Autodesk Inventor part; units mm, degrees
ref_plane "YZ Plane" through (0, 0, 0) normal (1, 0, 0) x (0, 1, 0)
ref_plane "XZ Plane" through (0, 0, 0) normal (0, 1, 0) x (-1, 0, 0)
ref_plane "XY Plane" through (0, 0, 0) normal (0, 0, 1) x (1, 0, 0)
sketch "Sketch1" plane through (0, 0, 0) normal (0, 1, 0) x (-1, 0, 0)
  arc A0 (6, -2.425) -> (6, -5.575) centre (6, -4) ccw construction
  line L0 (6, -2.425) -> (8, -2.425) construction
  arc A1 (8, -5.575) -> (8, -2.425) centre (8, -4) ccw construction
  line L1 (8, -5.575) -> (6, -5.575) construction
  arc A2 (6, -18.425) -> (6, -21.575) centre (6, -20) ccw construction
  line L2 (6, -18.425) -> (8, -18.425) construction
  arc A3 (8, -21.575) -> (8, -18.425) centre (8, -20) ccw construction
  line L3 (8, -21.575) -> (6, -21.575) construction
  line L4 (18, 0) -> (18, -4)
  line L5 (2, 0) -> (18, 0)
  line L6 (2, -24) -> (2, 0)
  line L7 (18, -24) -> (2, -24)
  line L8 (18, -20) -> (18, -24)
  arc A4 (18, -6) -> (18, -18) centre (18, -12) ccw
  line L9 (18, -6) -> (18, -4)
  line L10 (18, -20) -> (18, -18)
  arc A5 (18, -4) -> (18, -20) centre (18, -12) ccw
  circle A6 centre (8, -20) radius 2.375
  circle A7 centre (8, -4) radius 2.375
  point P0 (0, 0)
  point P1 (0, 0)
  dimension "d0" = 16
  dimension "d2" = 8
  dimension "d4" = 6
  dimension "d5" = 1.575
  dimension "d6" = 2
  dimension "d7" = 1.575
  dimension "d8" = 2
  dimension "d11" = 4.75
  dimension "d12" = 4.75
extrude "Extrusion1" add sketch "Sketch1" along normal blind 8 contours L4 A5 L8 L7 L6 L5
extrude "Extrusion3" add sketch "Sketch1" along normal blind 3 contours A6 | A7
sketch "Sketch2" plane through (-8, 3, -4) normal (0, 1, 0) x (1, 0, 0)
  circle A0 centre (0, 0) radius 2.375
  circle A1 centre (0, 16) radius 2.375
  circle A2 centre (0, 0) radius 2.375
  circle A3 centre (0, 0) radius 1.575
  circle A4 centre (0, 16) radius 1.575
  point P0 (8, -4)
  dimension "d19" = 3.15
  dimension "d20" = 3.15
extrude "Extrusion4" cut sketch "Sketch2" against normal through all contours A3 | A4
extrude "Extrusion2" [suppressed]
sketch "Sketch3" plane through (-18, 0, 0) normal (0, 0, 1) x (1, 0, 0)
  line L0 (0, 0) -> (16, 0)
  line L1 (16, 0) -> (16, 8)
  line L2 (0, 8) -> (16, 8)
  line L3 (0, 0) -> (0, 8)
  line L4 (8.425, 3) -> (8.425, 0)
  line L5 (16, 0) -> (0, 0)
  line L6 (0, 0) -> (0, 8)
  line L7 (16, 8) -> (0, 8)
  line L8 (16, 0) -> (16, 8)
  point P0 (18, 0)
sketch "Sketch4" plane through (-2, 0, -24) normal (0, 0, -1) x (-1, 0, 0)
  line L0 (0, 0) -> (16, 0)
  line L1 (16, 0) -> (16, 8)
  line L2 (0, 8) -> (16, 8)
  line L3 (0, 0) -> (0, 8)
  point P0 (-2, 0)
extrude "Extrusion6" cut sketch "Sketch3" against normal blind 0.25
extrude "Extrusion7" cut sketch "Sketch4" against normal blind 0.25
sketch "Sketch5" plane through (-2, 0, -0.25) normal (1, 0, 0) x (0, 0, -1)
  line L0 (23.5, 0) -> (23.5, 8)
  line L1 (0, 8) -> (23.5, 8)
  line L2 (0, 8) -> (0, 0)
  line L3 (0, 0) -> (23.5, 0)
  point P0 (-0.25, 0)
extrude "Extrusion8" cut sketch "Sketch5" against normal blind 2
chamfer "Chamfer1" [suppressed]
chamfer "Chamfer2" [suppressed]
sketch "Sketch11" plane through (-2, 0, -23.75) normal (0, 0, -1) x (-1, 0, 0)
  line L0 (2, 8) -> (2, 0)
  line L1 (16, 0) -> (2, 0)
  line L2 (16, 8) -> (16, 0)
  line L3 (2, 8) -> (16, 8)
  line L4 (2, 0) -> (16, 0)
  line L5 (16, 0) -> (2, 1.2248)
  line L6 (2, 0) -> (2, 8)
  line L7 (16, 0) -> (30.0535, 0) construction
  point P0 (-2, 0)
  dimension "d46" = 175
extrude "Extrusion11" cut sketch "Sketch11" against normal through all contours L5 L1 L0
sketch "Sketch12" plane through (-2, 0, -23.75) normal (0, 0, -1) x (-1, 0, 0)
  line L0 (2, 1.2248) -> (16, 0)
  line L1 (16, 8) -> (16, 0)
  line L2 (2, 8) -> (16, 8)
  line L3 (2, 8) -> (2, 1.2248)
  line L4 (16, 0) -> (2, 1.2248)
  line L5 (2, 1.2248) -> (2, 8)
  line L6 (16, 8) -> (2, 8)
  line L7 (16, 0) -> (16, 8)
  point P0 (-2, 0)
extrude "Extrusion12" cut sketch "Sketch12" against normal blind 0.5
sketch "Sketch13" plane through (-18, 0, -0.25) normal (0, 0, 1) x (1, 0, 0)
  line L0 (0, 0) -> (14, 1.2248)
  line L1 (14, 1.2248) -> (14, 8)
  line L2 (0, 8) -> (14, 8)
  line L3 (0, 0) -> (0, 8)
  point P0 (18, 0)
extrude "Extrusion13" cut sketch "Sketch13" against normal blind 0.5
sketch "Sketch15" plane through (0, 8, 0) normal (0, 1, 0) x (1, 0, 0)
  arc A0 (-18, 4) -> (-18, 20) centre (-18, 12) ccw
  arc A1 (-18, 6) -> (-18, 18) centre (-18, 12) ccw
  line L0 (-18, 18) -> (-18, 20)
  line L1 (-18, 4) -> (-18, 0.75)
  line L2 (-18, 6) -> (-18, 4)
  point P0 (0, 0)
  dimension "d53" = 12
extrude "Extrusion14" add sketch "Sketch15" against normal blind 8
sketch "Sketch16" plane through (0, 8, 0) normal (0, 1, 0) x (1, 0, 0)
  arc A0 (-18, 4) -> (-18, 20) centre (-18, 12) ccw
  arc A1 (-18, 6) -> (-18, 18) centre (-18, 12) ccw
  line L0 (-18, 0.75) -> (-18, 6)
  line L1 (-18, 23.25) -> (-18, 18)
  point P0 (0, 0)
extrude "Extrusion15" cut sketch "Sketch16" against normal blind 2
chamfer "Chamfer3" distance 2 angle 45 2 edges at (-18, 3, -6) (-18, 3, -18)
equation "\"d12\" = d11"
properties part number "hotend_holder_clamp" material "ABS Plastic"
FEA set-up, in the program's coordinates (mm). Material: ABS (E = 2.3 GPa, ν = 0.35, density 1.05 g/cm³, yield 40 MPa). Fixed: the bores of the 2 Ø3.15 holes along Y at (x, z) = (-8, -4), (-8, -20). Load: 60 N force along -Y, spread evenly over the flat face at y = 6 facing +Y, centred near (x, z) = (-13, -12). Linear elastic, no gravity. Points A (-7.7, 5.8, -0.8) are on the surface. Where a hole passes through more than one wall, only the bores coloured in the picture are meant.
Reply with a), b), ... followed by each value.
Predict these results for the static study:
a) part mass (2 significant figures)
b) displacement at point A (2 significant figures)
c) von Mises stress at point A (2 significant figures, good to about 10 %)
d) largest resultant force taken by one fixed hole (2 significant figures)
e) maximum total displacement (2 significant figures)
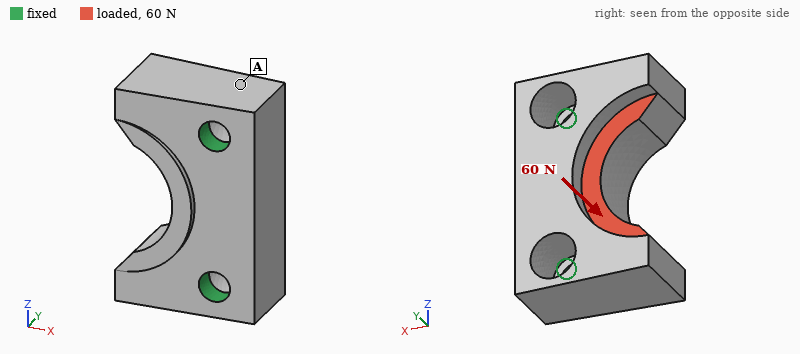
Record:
a) 1.7 g
b) 17 µm
c) 2.9 MPa
d) 32 N
e) 59 µm
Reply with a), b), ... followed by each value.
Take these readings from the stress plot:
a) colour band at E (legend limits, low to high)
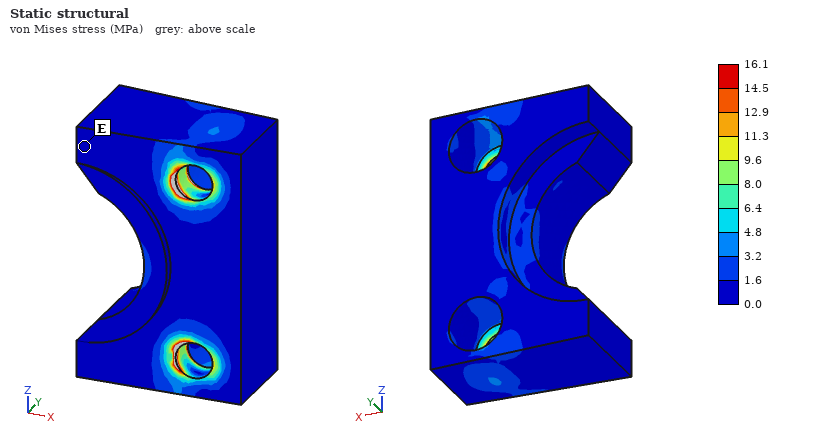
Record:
a) 0.0 to 1.6 MPa
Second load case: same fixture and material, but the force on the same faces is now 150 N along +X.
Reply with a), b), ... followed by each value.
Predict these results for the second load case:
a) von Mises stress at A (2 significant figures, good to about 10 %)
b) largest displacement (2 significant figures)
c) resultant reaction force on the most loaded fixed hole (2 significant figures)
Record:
a) 6.3 MPa
b) 0.12 mm
c) 76 N
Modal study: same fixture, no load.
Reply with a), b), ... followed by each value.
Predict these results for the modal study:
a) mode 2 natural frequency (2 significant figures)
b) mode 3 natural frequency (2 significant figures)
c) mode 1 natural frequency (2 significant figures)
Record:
a) 9200 Hz
b) 12 kHz
c) 5900 Hz
